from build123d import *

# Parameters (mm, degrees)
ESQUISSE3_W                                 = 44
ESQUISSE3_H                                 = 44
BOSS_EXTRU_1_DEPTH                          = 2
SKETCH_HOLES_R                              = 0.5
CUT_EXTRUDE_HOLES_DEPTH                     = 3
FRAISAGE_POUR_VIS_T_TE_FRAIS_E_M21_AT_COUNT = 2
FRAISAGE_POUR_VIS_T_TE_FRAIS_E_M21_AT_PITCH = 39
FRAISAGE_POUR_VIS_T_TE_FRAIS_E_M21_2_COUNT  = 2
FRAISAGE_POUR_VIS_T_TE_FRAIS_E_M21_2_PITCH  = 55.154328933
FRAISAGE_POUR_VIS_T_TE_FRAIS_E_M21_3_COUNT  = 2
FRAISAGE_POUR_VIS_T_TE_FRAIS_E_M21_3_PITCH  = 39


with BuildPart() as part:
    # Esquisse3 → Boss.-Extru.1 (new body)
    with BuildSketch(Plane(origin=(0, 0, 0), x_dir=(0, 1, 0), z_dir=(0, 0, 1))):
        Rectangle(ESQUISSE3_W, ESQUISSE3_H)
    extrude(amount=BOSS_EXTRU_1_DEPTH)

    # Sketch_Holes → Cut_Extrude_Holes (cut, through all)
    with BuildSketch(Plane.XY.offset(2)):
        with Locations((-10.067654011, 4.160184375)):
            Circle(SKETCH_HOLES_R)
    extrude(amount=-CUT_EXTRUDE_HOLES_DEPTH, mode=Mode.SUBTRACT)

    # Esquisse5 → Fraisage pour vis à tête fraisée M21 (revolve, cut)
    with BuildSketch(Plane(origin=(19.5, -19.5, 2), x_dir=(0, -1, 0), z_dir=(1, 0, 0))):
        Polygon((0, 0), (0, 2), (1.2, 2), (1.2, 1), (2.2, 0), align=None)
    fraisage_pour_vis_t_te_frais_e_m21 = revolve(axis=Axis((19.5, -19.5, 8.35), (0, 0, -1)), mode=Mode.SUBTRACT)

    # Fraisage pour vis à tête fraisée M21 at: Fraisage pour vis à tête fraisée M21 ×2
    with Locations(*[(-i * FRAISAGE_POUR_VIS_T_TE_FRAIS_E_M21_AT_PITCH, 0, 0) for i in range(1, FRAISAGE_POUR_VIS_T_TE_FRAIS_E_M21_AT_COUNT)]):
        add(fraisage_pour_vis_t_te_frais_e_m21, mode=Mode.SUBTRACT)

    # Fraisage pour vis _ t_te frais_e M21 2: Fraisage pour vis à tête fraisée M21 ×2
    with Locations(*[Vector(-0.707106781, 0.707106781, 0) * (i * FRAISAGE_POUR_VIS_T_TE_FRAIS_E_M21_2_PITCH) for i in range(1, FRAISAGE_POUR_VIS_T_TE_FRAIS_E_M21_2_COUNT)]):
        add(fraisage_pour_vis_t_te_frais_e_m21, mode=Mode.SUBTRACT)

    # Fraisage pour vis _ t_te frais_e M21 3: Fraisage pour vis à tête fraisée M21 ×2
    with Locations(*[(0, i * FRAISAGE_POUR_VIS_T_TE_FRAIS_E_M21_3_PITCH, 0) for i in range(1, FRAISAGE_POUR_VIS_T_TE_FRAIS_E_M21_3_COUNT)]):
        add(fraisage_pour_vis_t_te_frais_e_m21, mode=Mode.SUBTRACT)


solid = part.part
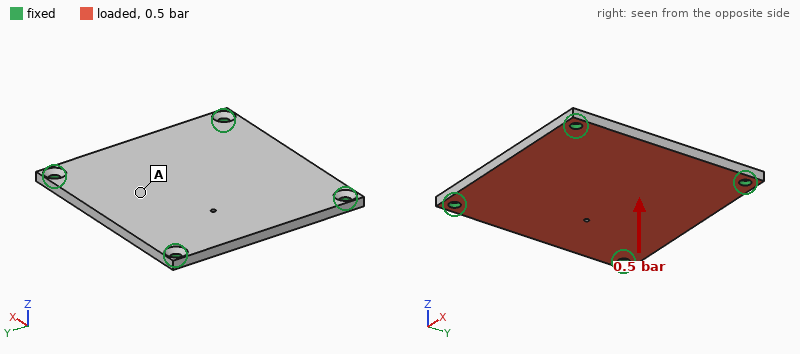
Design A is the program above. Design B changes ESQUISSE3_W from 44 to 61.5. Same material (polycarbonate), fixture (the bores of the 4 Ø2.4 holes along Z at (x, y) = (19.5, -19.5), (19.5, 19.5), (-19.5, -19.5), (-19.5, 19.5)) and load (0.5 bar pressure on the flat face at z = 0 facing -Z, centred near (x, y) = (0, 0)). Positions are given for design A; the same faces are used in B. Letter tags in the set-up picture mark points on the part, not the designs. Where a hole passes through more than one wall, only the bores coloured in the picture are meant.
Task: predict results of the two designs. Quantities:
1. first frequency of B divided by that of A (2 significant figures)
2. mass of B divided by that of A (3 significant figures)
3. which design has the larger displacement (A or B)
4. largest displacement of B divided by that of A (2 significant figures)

1.0
1.40
A
0.90
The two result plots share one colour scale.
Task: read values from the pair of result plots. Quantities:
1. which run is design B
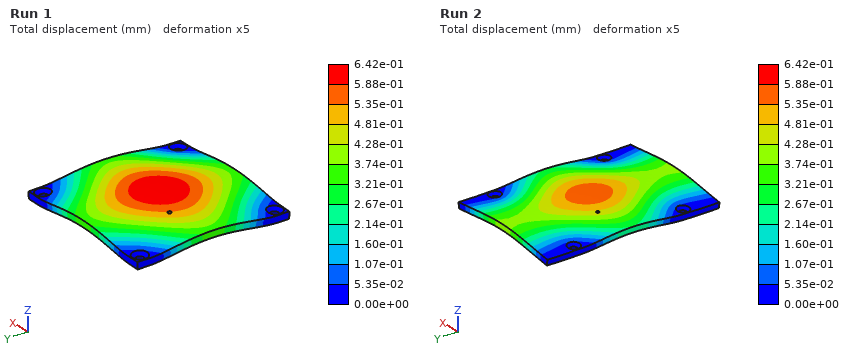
Run 2
